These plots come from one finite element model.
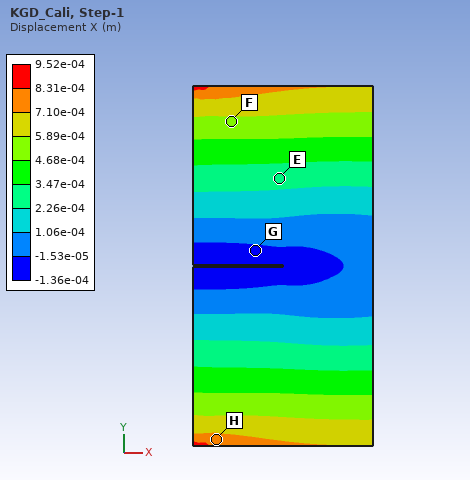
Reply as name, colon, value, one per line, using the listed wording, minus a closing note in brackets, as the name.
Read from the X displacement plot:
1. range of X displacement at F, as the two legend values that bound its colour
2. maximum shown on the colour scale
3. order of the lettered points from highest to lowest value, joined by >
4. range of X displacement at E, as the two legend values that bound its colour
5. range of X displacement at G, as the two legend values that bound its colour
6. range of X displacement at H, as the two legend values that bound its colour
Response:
range of X displacement at F, as the two legend values that bound its colour: 4.68e-04 to 5.89e-04 m
maximum shown on the colour scale: 9.52e-04 m
order of the lettered points from highest to lowest value, joined by >: H > F > E > G
range of X displacement at E, as the two legend values that bound its colour: 2.26e-04 to 3.47e-04 m
range of X displacement at G, as the two legend values that bound its colour: -1.36e-04 to -1.53e-05 m
range of X displacement at H, as the two legend values that bound its colour: 7.10e-04 to 8.31e-04 m
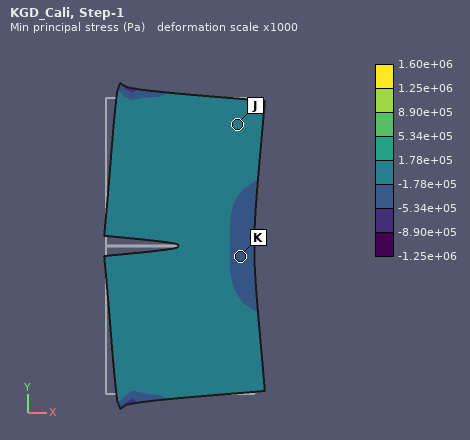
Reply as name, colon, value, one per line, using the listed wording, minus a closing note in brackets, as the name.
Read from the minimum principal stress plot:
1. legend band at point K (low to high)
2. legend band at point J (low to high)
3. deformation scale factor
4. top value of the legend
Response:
legend band at point K: -5.34e+05 to -1.78e+05 Pa
legend band at point J: -1.78e+05 to 1.78e+05 Pa
deformation scale factor: 1000
top value of the legend: 1.60e+06 Pa
